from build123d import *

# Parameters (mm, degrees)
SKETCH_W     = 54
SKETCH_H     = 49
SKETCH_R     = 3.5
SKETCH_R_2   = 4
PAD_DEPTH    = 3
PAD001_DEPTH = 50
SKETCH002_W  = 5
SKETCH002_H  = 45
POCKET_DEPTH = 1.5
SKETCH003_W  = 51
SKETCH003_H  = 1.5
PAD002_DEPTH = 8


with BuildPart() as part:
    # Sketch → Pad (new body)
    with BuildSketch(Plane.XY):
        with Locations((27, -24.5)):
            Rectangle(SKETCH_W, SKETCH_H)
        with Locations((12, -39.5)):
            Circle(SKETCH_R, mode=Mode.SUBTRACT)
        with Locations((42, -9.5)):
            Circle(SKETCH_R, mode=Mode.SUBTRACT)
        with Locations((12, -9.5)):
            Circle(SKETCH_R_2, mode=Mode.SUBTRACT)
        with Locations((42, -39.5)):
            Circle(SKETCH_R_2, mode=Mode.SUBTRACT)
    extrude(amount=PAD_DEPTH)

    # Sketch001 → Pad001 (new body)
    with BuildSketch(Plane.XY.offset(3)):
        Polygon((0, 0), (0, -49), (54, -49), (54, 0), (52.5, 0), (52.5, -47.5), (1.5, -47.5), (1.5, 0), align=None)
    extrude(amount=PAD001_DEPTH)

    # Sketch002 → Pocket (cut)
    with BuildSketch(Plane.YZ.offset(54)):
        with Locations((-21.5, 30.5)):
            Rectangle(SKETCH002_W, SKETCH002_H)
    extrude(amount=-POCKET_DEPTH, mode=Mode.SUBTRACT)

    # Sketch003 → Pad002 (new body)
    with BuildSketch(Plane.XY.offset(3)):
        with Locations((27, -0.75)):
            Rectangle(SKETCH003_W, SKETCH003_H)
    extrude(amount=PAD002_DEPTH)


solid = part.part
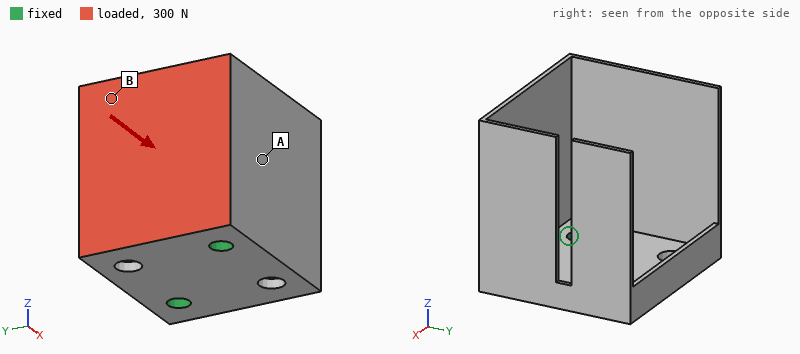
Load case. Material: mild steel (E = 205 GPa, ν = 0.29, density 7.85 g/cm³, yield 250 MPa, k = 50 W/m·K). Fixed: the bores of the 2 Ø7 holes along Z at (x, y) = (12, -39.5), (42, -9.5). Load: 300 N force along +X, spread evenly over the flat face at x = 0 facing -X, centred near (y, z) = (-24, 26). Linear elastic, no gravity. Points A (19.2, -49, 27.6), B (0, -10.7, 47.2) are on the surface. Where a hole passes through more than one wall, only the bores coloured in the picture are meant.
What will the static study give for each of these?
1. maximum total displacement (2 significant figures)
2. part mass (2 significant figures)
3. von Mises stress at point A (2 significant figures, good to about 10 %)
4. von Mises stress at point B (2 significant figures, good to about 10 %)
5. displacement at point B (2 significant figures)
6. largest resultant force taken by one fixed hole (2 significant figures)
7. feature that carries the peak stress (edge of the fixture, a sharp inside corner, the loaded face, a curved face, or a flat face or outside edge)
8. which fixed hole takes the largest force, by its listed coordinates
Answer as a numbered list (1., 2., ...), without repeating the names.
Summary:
1. 0.55 mm
2. 150 g
3. 18 MPa
4. 49 MPa
5. 0.41 mm
6. 190 N
7. the loaded face
8. (12, -39.5)
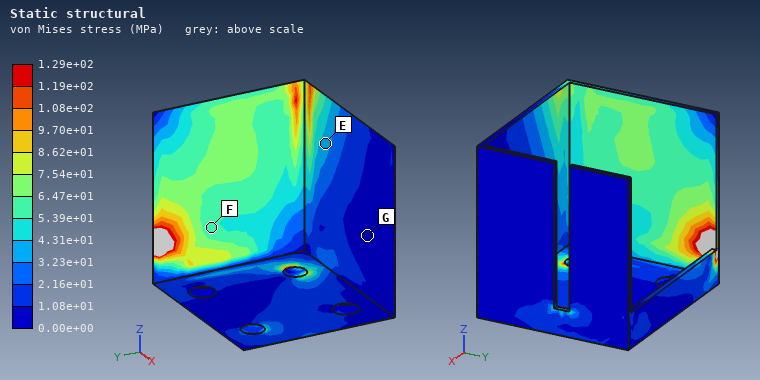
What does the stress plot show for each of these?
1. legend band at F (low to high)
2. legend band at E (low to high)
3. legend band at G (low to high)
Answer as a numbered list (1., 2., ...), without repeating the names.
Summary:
1. 5.39e+01 to 6.47e+01 MPa
2. 3.23e+01 to 4.31e+01 MPa
3. 0.00e+00 to 1.08e+01 MPa
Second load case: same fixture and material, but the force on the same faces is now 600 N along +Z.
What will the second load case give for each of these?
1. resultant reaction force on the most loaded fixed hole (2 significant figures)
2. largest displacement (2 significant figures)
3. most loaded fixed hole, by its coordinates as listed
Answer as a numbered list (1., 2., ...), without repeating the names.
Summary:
1. 520 N
2. 0.14 mm
3. (12, -39.5)
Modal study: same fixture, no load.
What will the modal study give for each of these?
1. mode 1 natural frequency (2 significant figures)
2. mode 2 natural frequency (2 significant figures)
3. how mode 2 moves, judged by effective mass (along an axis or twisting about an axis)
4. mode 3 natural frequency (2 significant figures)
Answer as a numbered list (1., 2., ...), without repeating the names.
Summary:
1. 560 Hz
2. 910 Hz
3. along X
4. 1200 Hz
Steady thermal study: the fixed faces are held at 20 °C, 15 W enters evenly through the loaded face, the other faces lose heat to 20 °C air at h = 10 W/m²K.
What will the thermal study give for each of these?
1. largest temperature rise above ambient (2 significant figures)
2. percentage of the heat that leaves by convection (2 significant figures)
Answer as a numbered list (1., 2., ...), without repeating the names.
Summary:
1. 83 K
2. 24 %
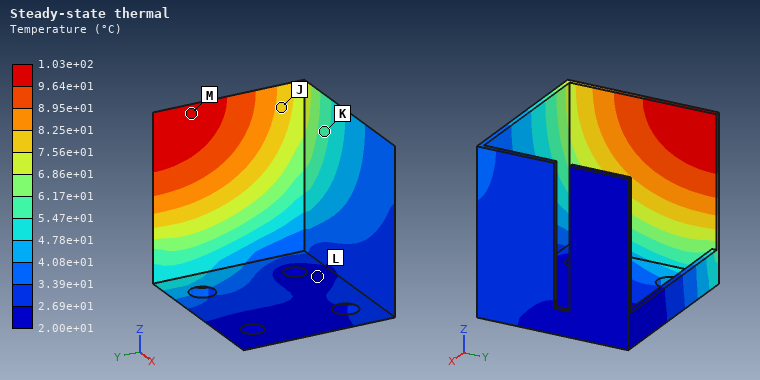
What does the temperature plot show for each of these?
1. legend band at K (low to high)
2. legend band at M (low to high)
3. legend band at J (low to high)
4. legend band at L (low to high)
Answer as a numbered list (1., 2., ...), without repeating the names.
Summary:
1. 5.47e+01 to 6.17e+01 °C
2. 9.64e+01 to 1.03e+02 °C
3. 7.56e+01 to 8.25e+01 °C
4. 2.00e+01 to 2.69e+01 °C
